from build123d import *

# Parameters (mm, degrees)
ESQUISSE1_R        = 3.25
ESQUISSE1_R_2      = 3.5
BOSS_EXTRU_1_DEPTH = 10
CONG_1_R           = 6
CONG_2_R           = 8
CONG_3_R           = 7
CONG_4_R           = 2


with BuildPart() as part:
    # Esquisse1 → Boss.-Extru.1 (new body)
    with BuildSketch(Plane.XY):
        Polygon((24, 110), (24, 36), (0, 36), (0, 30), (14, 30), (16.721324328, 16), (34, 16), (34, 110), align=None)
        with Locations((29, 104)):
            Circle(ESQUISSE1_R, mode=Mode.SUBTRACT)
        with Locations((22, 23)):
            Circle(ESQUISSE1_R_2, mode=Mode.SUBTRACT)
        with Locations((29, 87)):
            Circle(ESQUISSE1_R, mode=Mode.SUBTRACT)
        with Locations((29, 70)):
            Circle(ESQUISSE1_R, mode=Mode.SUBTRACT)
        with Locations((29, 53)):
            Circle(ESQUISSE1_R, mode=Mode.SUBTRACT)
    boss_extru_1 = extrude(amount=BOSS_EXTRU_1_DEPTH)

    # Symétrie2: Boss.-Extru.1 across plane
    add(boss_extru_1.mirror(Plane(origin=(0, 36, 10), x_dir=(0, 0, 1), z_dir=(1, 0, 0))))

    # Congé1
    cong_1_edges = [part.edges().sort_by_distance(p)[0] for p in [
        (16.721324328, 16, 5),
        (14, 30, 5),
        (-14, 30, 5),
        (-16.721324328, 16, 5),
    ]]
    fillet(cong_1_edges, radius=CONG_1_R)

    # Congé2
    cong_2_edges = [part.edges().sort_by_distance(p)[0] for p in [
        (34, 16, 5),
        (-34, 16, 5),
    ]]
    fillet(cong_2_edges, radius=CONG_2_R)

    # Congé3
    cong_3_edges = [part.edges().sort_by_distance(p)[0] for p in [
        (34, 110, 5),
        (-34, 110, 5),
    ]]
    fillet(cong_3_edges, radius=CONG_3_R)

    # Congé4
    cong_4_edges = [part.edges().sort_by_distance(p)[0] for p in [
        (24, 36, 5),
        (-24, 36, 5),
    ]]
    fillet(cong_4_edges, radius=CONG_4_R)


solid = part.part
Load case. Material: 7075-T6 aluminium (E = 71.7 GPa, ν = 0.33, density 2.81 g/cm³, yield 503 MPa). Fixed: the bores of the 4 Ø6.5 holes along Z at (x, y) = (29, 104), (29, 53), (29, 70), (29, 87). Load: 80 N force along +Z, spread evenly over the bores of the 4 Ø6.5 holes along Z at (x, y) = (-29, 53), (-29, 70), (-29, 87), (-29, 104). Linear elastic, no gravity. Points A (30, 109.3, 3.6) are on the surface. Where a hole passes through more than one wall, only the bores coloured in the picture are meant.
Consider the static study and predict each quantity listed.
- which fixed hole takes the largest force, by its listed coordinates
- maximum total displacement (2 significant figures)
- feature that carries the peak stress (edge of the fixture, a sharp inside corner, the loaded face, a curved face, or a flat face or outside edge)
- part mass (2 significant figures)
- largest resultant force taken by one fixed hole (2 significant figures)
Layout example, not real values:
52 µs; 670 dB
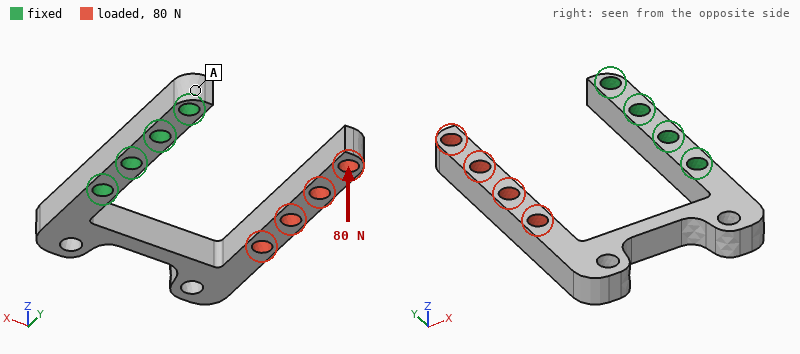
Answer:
(29, 53); 1.1 mm; a flat face or outside edge; 57 g; 78 N
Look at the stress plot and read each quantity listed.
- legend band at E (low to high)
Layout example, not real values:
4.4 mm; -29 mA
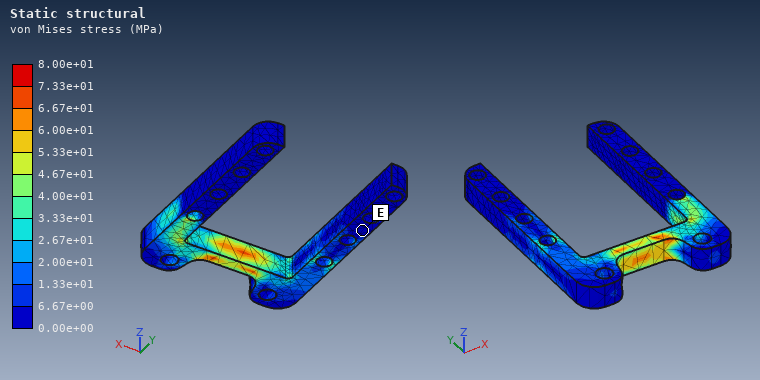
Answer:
0.00e+00 to 6.67e+00 MPa
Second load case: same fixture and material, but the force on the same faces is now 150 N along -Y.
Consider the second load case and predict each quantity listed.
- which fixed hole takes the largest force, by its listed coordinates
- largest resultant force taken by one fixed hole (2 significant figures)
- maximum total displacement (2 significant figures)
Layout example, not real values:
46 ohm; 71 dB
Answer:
(29, 53); 150 N; 1.1 mm
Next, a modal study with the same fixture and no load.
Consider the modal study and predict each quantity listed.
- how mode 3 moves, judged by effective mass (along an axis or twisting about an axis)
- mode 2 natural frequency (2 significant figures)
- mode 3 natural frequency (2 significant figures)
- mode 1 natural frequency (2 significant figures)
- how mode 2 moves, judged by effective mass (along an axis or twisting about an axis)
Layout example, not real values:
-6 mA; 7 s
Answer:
along Z; 420 Hz; 910 Hz; 390 Hz; along Z
